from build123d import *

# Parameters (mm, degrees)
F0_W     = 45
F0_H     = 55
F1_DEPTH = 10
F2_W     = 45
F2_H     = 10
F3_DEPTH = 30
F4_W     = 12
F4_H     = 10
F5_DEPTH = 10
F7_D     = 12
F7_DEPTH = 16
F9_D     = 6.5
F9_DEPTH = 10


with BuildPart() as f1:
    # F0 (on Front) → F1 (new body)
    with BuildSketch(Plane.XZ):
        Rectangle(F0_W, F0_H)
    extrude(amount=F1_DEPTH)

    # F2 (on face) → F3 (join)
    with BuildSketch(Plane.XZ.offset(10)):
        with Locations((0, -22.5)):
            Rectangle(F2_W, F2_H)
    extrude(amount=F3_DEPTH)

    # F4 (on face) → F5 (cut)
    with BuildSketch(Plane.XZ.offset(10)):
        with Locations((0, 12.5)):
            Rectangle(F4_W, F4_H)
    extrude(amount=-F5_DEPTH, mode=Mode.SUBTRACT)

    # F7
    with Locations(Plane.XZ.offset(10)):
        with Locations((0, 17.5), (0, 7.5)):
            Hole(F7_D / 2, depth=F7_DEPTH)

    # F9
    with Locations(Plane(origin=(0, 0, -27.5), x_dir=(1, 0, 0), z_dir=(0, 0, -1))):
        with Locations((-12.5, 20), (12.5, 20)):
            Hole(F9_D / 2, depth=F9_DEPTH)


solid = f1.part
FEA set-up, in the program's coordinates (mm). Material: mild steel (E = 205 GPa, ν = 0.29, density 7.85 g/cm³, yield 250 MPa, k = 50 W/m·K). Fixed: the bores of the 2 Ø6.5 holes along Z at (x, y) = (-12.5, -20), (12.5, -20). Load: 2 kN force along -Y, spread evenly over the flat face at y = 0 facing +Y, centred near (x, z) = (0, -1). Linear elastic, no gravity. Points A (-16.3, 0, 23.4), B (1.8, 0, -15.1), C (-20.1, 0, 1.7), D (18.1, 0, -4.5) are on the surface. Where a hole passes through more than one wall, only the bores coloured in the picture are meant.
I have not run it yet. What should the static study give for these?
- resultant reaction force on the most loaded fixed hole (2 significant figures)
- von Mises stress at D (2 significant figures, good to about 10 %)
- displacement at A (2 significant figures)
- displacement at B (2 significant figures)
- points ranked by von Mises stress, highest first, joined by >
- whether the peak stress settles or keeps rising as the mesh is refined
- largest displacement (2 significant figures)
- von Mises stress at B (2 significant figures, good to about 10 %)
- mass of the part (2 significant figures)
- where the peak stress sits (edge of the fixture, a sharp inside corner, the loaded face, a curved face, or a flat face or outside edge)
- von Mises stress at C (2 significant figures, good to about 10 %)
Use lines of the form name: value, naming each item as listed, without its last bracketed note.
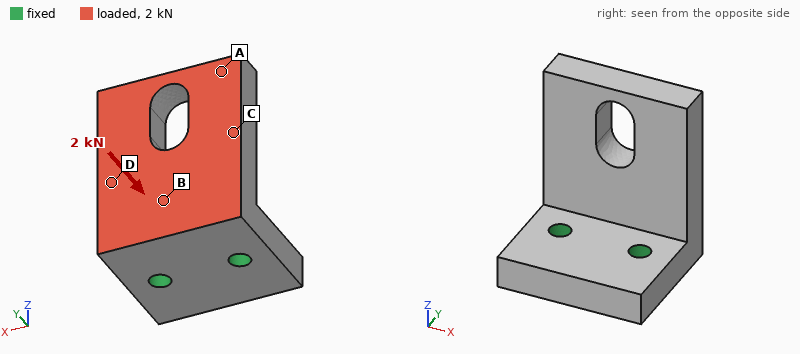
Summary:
resultant reaction force on the most loaded fixed hole: 1.0 kN
von Mises stress at D: 25 MPa
displacement at A: 61 µm
displacement at B: 13 µm
points ranked by von Mises stress, highest first, joined by >: B > D > C > A
whether the peak stress settles or keeps rising as the mesh is refined: keeps rising
largest displacement: 68 µm
von Mises stress at B: 38 MPa
mass of the part: 280 g
where the peak stress sits: edge of the fixture
von Mises stress at C: 18 MPa
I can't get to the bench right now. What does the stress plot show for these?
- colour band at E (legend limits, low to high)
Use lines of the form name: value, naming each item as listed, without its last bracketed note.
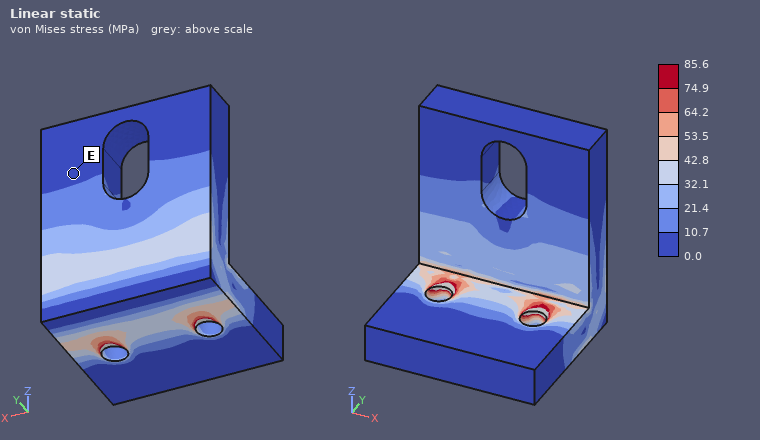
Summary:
colour band at E: 0.0 to 10.7 MPa
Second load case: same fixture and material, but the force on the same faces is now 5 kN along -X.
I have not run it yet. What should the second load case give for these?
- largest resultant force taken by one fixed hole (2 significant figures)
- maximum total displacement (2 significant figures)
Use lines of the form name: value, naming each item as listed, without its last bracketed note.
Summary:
largest resultant force taken by one fixed hole: 5.3 kN
maximum total displacement: 35 µm
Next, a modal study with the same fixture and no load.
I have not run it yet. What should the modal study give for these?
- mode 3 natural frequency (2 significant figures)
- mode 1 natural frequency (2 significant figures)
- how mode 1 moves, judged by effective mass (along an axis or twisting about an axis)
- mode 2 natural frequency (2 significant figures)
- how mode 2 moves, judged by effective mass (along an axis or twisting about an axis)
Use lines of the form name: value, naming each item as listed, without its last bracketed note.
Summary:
mode 3 natural frequency: 7000 Hz
mode 1 natural frequency: 2500 Hz
how mode 1 moves, judged by effective mass: along Y
mode 2 natural frequency: 5100 Hz
how mode 2 moves, judged by effective mass: along X
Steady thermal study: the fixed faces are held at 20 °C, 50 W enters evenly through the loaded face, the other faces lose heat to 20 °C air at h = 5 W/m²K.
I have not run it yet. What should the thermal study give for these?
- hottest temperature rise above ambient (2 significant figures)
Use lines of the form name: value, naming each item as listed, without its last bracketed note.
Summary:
hottest temperature rise above ambient: 76 K
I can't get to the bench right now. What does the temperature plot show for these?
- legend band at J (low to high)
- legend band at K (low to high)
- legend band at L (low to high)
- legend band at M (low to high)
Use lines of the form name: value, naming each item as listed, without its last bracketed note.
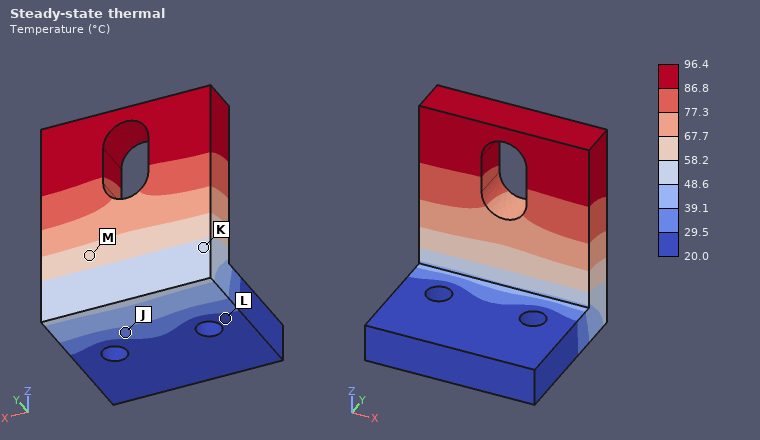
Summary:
legend band at J: 29.5 to 39.1 °C
legend band at K: 48.6 to 58.2 °C
legend band at L: 20.0 to 29.5 °C
legend band at M: 58.2 to 67.7 °C
